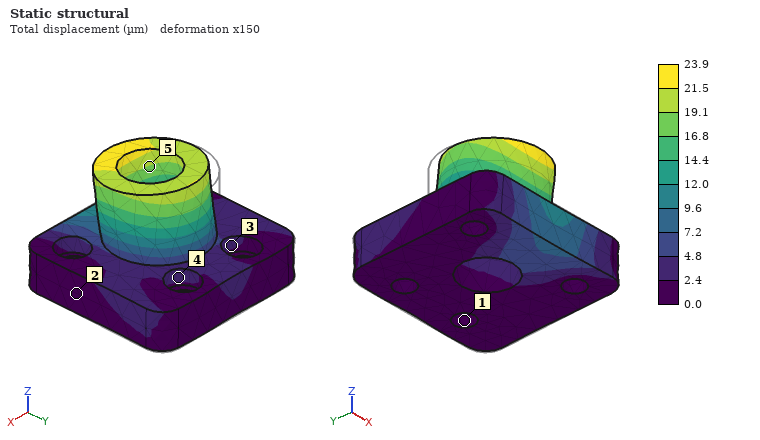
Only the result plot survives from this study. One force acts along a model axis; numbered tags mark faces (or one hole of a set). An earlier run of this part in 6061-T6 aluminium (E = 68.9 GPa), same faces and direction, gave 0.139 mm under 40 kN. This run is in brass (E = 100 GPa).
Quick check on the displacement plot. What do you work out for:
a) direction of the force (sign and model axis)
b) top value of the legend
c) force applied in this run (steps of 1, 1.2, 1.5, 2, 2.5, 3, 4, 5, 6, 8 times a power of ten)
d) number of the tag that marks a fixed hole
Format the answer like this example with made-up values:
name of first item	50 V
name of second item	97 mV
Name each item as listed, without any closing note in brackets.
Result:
direction of the force	-Y
top value of the legend	23.9 µm
force applied in this run	10 kN
number of the tag that marks a fixed hole	1
